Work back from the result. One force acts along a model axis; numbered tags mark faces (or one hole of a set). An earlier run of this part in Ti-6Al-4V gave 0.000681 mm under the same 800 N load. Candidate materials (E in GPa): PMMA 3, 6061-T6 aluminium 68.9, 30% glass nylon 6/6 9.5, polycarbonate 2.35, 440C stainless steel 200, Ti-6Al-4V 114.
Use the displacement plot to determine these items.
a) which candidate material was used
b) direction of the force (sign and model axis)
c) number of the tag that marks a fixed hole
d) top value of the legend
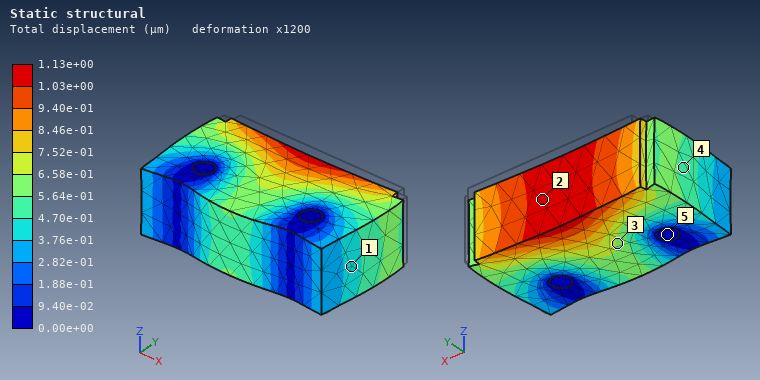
6061-T6 aluminium
-Y
5
1.13e+00 µm
